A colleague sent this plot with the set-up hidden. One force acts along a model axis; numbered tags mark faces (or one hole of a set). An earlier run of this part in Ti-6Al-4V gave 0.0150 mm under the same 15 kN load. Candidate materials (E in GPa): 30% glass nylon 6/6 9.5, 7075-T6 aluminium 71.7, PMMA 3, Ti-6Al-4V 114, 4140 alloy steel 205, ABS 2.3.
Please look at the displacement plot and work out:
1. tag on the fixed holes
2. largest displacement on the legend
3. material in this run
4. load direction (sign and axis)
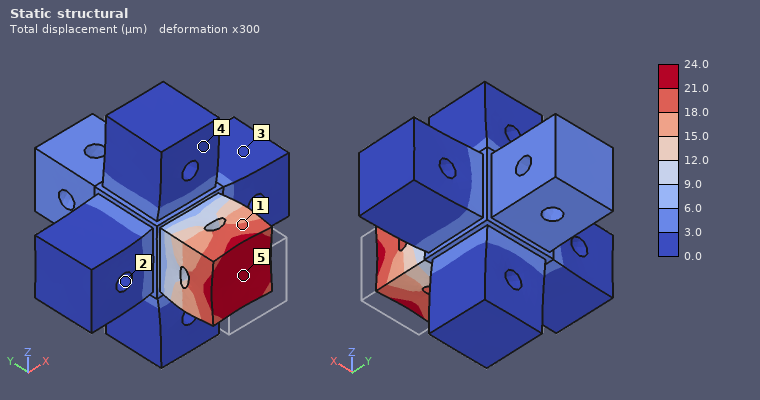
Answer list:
2
24.0 µm
7075-T6 aluminium
+Y
